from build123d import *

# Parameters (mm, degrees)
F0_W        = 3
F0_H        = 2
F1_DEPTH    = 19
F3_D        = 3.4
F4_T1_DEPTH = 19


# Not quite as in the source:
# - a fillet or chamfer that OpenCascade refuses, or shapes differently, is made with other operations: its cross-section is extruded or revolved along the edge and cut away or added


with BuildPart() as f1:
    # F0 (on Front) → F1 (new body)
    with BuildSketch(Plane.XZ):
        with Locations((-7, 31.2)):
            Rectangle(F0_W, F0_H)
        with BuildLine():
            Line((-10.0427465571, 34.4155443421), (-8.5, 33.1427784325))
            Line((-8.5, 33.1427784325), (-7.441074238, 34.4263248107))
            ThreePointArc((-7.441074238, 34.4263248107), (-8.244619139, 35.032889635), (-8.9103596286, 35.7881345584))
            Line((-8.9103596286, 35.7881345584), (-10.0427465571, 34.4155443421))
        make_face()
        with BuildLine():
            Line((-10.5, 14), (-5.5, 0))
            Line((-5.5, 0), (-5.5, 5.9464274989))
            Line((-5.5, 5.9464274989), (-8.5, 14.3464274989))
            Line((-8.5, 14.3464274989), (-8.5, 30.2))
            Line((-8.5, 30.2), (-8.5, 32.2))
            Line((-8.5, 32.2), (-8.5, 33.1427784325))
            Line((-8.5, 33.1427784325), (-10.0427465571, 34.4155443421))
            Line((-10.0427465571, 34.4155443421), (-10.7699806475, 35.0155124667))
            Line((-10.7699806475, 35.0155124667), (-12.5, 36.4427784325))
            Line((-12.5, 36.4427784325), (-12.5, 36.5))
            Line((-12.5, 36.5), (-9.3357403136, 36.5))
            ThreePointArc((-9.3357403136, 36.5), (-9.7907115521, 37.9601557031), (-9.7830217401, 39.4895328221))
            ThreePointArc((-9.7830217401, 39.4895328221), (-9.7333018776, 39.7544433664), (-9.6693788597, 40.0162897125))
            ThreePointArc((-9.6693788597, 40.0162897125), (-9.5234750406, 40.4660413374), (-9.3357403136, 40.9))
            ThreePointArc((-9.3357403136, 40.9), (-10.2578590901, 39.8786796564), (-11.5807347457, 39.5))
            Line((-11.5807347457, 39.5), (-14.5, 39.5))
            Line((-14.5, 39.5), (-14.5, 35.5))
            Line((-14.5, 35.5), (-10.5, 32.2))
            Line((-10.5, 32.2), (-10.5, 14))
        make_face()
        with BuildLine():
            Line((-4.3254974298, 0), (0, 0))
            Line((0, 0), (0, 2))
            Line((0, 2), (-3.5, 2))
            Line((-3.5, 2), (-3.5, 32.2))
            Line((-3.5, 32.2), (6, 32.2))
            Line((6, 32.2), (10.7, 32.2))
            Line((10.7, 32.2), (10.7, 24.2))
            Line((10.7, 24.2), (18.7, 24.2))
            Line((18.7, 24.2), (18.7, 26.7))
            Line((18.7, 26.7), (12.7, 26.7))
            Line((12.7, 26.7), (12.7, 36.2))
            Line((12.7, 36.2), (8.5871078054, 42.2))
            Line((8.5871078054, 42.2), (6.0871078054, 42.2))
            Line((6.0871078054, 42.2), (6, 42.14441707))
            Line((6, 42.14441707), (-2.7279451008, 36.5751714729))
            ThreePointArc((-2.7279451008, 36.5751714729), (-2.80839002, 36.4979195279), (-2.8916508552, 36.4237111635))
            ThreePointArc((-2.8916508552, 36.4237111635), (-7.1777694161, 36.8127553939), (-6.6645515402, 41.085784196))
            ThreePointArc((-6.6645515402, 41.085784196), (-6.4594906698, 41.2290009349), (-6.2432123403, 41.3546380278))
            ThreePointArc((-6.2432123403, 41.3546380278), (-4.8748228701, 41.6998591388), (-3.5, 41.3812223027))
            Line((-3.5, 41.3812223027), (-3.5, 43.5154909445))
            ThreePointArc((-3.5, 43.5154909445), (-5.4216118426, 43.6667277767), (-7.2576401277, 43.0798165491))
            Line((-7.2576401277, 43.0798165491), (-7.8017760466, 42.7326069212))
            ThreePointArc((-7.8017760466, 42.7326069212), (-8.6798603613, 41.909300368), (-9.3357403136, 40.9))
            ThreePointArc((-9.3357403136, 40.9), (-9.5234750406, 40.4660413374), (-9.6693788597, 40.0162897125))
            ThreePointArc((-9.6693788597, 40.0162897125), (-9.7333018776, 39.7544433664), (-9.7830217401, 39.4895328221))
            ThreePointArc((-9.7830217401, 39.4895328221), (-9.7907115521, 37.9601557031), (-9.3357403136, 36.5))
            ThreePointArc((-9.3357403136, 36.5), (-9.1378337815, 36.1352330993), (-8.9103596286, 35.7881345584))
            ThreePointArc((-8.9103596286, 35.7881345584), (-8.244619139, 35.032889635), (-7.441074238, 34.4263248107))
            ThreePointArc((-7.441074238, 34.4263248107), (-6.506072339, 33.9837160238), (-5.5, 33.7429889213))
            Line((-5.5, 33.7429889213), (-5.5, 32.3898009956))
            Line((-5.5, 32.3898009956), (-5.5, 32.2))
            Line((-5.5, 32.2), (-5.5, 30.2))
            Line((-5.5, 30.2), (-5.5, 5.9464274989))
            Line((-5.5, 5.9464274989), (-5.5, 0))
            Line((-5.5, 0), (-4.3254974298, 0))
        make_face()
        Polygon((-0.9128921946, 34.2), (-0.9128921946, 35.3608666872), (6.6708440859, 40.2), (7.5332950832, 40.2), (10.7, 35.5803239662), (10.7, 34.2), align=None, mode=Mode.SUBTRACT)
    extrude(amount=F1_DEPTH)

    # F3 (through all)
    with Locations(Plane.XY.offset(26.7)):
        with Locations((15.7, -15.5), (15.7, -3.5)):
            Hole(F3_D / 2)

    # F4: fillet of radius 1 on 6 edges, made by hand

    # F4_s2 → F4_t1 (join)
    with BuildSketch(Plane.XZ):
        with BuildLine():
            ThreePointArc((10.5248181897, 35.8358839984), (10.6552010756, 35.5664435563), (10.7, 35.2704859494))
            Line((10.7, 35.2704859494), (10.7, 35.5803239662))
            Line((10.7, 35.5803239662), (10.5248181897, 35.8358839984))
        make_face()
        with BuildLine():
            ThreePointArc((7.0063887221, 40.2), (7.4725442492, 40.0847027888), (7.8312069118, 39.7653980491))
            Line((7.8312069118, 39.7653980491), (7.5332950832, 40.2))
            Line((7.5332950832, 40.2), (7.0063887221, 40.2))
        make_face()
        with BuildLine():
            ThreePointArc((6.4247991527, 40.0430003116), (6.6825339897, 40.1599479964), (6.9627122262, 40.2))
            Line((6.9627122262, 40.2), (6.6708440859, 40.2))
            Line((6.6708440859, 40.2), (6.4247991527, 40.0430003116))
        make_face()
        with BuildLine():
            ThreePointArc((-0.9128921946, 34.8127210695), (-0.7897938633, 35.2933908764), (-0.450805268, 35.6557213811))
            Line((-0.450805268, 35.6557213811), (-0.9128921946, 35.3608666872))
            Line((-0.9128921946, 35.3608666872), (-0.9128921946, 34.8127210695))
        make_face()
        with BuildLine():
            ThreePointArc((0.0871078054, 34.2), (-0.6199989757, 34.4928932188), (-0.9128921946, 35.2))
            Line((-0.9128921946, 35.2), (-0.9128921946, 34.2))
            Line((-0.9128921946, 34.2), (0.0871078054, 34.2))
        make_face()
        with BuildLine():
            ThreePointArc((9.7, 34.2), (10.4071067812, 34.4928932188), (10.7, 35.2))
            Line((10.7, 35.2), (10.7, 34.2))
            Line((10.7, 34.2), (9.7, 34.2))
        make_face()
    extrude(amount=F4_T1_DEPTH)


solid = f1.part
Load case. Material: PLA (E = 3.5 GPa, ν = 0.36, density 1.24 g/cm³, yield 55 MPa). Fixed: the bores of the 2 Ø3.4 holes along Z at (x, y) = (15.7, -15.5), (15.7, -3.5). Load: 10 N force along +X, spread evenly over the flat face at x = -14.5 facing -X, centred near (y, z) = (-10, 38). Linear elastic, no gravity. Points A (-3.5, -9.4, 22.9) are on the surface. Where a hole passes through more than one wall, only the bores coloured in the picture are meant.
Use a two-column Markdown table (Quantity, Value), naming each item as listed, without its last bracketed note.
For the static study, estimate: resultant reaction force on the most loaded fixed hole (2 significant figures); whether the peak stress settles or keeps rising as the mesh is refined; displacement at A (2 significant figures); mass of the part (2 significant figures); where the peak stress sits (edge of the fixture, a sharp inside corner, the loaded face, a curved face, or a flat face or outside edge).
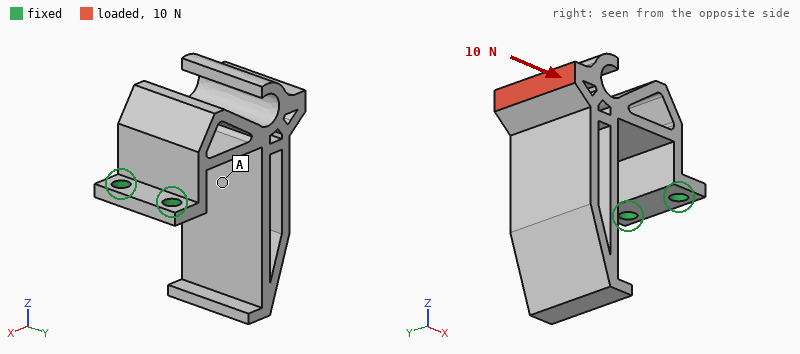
| Quantity | Value |
|---|---|
| resultant reaction force on the most loaded fixed hole | 5.1 N |
| whether the peak stress settles or keeps rising as the mesh is refined | keeps rising |
| displacement at A | 0.28 mm |
| mass of the part | 7.2 g |
| where the peak stress sits | edge of the fixture |
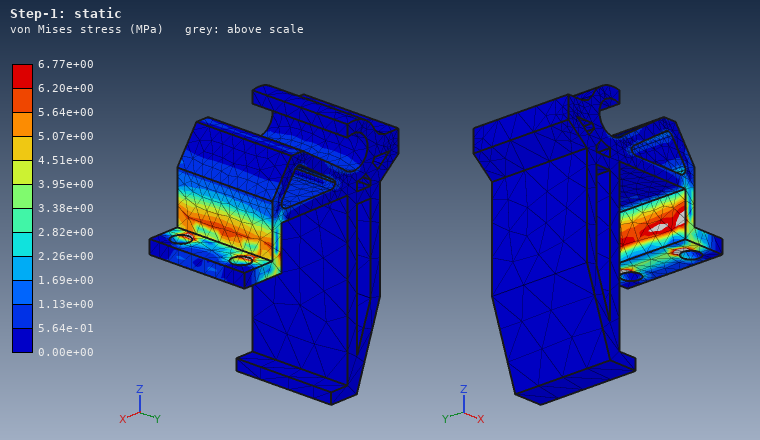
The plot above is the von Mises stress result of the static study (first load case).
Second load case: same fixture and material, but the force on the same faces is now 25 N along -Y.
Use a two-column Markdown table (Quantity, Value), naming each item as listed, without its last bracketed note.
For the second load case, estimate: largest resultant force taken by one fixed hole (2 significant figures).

| Quantity | Value |
|---|---|
| largest resultant force taken by one fixed hole | 60 N |
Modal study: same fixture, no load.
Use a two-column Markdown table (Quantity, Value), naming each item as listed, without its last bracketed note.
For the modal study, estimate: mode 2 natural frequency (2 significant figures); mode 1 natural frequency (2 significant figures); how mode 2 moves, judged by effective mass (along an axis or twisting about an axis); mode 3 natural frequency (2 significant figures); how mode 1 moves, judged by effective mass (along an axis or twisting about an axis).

| Quantity | Value |
|---|---|
| mode 2 natural frequency | 540 Hz |
| mode 1 natural frequency | 200 Hz |
| how mode 2 moves, judged by effective mass | along Y |
| mode 3 natural frequency | 790 Hz |
| how mode 1 moves, judged by effective mass | along Z |
